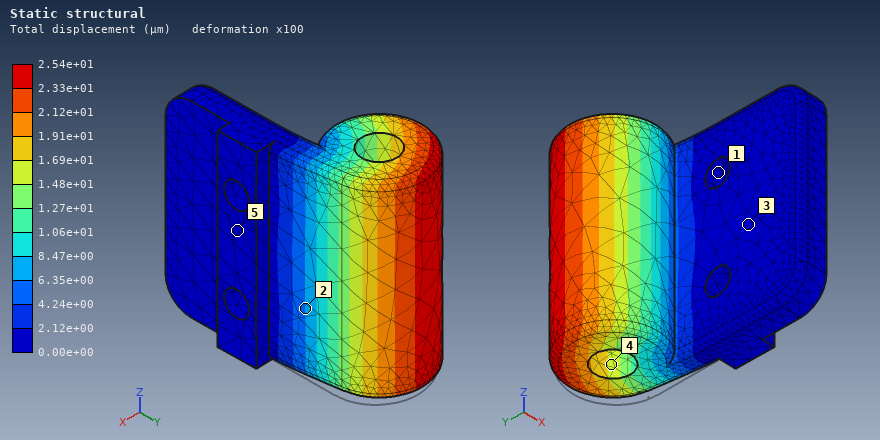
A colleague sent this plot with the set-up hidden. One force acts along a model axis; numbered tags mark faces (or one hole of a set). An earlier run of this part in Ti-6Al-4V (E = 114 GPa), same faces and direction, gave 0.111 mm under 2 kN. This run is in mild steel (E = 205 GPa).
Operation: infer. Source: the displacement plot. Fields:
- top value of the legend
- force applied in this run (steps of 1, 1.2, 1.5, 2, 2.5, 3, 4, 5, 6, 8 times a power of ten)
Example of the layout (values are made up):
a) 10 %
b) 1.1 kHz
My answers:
a) 2.54e+01 µm
b) 800 N
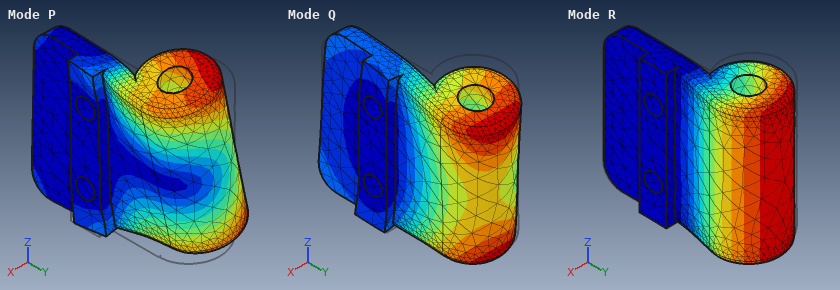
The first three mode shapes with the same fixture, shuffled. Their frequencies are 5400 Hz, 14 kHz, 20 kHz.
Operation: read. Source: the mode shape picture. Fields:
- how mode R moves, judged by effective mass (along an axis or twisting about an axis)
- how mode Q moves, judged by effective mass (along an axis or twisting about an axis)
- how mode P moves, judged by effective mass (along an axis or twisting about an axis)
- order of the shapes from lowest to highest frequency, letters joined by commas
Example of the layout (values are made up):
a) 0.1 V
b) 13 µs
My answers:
a) along X
b) along Z
c) along Z
d) R, P, Q
